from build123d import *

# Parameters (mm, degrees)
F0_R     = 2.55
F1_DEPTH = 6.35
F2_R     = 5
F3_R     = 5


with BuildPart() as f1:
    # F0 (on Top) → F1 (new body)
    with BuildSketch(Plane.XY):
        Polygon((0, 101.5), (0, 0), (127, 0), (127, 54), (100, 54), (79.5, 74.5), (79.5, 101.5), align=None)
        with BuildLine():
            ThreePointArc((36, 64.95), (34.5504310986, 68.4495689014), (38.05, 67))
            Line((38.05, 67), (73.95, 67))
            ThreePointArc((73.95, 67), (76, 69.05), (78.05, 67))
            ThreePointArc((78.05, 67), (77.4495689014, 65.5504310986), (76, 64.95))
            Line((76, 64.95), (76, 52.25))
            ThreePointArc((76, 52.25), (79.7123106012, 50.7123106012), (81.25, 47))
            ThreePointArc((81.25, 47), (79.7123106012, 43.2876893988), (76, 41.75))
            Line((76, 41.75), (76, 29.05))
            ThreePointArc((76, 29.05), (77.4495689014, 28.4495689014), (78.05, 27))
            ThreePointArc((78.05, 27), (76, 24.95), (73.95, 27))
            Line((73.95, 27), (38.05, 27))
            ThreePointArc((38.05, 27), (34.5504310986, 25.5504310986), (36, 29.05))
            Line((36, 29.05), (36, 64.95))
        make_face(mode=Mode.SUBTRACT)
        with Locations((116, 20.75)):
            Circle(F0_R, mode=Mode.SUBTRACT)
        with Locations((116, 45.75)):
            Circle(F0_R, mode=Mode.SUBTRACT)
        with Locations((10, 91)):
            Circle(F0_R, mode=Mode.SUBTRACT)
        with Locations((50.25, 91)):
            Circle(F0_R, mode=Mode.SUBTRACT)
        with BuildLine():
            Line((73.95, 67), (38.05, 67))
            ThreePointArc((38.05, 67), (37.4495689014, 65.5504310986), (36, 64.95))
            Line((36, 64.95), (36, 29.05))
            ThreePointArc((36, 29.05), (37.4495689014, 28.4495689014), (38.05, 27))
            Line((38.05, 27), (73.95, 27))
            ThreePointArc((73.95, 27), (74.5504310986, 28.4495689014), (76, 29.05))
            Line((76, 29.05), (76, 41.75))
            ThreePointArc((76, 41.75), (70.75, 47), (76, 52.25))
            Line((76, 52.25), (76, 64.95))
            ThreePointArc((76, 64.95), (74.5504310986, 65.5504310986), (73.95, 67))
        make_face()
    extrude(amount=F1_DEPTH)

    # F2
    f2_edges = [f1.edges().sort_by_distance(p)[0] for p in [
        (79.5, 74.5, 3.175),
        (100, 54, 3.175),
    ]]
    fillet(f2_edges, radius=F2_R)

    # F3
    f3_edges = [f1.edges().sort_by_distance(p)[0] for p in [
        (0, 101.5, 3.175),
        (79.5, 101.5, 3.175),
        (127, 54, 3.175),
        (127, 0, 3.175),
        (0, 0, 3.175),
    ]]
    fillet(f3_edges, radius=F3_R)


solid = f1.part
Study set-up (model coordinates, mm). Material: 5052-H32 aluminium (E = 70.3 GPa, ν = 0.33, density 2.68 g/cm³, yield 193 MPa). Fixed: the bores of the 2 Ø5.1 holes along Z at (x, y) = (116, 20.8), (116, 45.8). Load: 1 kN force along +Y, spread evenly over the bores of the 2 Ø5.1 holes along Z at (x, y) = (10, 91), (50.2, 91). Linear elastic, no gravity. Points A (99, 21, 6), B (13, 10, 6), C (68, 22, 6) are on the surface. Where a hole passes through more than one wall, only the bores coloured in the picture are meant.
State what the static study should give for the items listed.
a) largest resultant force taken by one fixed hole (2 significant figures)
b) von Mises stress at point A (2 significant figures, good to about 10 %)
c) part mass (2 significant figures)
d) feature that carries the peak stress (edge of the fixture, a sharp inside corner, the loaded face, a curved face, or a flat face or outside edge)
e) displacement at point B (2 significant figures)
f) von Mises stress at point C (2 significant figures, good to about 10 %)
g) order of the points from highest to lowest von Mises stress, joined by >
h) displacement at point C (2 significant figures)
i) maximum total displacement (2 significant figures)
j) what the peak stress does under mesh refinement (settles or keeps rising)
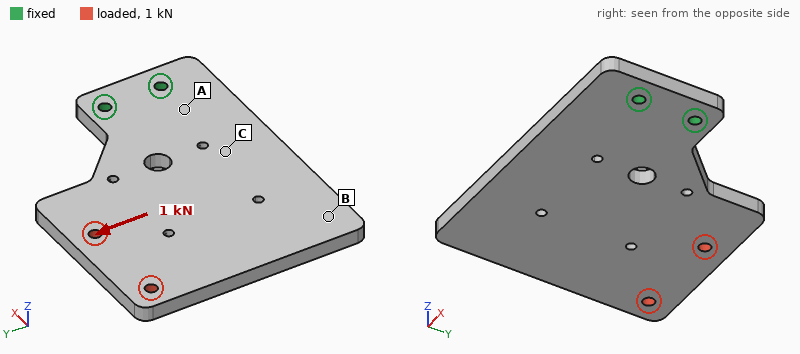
3.1 kN
16 MPa
180 g
edge of the fixture
0.083 mm
7.7 MPa
A > C > B
0.034 mm
0.11 mm
keeps rising
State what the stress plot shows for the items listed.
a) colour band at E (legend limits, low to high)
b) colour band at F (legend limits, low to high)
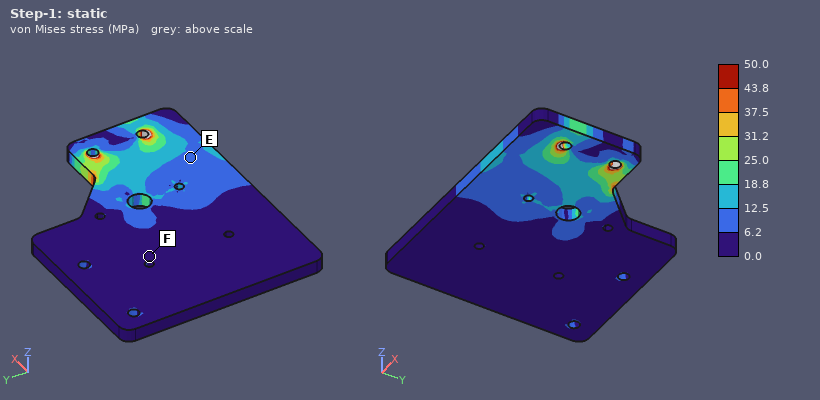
6.2 to 12.5 MPa
0.0 to 6.2 MPa
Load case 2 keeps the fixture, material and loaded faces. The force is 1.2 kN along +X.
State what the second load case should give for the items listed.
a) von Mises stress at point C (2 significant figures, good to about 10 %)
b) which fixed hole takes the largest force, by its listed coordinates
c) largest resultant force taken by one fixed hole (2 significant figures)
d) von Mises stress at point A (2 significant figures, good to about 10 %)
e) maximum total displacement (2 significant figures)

5.9 MPa
(116, 45.8)
3.1 kN
10 MPa
0.10 mm
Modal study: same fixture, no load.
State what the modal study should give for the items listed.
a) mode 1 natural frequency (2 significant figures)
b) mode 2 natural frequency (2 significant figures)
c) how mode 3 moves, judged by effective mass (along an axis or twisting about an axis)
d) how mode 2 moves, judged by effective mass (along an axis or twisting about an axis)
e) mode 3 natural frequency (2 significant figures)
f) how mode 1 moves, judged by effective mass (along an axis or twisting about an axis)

280 Hz
720 Hz
along Y
twisting about X
1600 Hz
along Z
